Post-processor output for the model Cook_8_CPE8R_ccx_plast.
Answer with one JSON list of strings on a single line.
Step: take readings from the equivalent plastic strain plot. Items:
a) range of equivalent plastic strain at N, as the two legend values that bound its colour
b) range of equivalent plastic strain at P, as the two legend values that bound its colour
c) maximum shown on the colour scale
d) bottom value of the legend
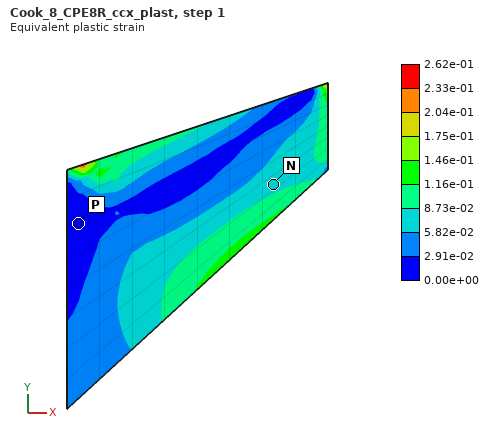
["5.82e-02 to 8.73e-02", "0.00e+00 to 2.91e-02", "2.62e-01", "0.00e+00"]
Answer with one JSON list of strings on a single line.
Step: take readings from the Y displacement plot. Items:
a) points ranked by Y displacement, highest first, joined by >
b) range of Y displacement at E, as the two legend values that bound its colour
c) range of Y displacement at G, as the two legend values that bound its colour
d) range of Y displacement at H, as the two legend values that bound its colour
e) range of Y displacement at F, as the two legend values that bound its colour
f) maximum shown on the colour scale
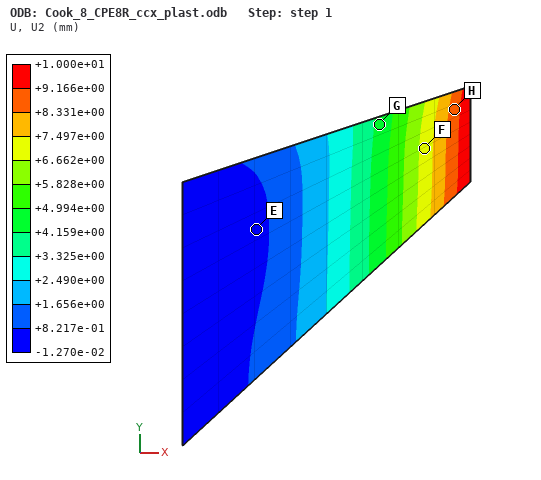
["H > F > G > E", "-1.270e-02 to +8.217e-01 mm", "+4.159e+00 to +4.994e+00 mm", "+8.331e+00 to +9.166e+00 mm", "+6.662e+00 to +7.497e+00 mm", "+1.000e+01 mm"]
